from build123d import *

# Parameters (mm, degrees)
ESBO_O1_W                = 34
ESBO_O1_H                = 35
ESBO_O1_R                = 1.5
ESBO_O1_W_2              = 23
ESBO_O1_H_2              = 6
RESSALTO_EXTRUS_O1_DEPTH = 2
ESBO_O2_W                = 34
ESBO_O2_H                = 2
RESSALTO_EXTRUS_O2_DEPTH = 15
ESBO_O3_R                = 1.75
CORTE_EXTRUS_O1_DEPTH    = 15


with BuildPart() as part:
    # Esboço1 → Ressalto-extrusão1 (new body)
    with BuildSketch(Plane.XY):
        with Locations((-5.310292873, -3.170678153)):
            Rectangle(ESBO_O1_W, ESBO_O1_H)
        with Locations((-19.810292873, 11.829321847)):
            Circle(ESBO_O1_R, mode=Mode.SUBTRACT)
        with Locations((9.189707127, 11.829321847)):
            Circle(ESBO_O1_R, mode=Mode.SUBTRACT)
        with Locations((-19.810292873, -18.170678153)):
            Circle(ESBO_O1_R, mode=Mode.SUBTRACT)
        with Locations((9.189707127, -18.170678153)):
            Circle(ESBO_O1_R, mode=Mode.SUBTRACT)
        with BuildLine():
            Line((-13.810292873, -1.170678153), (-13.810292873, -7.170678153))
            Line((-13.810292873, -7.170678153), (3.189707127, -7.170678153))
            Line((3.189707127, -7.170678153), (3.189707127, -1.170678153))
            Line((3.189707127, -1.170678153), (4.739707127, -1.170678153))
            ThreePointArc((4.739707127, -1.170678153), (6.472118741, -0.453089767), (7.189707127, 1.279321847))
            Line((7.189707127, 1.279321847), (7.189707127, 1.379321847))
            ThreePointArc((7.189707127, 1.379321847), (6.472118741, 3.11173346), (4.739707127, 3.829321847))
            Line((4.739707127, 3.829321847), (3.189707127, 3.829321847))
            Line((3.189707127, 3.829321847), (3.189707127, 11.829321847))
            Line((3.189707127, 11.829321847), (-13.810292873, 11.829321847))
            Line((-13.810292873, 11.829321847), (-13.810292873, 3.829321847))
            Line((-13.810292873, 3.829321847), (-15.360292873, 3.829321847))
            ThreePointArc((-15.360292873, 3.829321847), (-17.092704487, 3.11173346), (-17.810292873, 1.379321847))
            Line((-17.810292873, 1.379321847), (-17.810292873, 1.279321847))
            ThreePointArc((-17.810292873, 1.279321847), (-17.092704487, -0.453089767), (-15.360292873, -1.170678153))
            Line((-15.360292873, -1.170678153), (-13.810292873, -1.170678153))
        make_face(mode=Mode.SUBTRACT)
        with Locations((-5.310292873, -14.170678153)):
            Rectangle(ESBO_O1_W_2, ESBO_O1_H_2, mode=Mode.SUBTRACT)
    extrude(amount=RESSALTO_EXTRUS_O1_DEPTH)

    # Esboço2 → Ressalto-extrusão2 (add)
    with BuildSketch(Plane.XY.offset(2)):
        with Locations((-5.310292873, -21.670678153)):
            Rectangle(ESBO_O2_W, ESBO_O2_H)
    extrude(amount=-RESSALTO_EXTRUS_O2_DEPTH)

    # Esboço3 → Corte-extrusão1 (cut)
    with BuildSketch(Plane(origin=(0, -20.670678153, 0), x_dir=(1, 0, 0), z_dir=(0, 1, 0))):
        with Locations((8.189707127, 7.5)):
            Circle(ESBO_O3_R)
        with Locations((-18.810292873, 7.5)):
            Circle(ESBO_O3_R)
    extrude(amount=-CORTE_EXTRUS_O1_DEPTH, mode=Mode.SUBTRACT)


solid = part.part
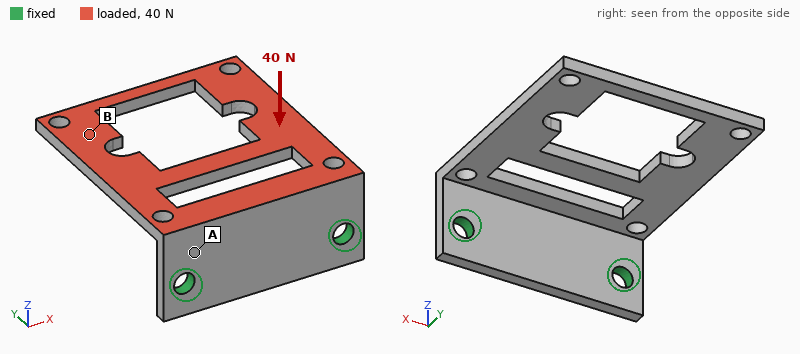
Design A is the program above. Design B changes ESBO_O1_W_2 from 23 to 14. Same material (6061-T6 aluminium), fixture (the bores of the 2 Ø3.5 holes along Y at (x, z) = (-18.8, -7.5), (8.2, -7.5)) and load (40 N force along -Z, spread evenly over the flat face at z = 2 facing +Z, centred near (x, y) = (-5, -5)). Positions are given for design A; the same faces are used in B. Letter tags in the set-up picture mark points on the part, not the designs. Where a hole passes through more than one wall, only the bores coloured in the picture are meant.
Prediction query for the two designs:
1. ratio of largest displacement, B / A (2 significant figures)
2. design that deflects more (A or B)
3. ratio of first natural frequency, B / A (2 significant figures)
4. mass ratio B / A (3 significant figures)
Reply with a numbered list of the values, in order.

1. 0.62
2. A
3. 1.2
4. 1.05
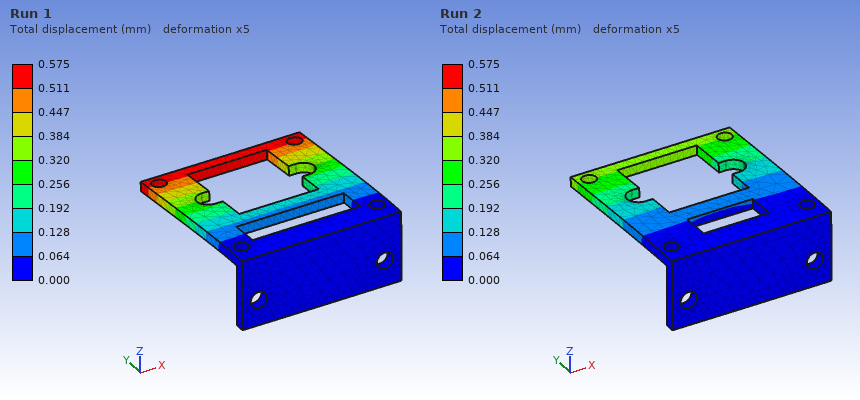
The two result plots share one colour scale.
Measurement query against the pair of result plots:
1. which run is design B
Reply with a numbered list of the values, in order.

1. Run 2
